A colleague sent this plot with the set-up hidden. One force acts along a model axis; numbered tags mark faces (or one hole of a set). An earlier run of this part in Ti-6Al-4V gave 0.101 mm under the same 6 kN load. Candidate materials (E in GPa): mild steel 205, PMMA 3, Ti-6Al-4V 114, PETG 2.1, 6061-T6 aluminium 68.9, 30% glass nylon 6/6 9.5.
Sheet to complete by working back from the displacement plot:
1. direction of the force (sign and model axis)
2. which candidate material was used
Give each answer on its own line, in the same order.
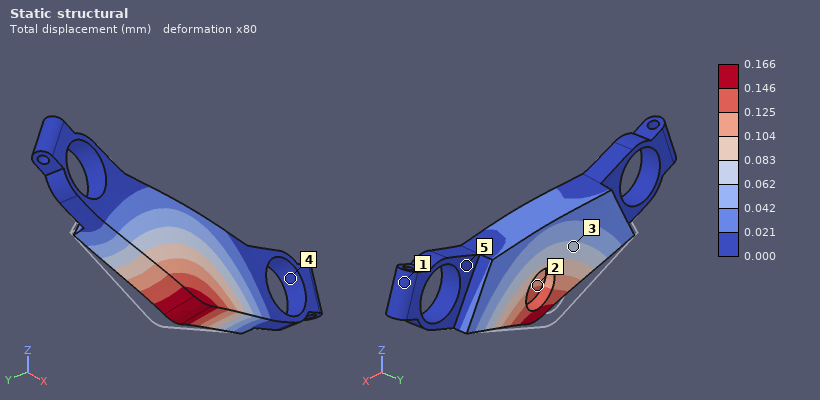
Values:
-Y
6061-T6 aluminium
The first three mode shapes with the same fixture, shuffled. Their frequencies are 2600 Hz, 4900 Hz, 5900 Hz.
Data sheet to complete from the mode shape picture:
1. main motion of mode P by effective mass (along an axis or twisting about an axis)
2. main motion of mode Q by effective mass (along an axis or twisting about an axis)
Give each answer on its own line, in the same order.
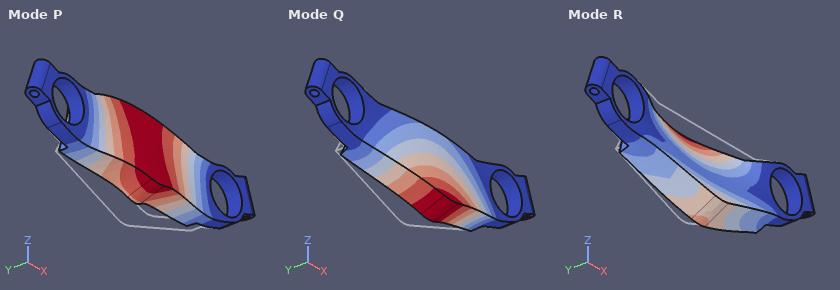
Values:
along Z
along Y
